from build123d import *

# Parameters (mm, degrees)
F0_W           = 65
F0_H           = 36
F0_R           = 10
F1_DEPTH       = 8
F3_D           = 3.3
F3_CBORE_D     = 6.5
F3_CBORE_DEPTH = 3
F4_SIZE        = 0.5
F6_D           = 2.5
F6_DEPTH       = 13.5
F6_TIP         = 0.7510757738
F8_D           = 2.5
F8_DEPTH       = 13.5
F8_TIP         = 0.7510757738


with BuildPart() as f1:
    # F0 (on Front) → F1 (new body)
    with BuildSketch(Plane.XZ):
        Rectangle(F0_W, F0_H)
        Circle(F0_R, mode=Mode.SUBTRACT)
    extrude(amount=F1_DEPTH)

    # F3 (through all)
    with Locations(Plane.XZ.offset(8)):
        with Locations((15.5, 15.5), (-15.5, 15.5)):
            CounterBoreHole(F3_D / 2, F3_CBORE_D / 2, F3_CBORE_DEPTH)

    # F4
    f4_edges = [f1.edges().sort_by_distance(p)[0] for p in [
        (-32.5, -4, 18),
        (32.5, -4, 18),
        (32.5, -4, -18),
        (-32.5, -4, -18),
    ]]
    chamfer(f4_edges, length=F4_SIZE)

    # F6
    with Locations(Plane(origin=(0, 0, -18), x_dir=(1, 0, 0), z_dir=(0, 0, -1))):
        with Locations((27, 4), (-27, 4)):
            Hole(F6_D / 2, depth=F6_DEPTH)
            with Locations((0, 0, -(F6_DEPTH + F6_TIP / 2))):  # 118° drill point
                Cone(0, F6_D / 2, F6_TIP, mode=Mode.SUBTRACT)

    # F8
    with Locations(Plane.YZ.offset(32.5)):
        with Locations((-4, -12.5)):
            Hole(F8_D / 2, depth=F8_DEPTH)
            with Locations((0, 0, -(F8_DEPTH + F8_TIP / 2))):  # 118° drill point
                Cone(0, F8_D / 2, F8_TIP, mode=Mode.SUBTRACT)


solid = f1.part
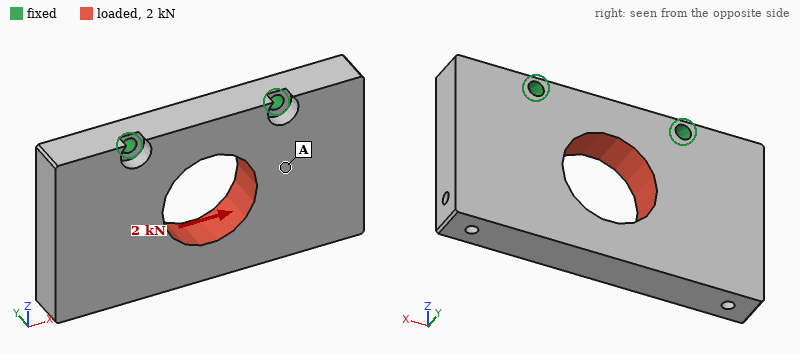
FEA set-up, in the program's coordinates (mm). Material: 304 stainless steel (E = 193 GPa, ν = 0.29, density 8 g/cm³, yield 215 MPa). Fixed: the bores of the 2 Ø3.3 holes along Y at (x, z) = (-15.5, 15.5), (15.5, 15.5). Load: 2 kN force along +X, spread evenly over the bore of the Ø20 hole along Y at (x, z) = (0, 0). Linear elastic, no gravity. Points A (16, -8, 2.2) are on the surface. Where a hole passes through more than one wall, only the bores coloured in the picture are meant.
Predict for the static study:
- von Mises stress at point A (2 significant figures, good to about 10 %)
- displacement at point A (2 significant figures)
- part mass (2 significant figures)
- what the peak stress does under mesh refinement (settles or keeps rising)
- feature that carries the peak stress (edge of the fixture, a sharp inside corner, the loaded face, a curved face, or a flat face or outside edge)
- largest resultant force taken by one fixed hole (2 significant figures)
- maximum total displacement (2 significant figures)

10 MPa
3.9 µm
130 g
keeps rising
edge of the fixture
1.3 kN
9.9 µm
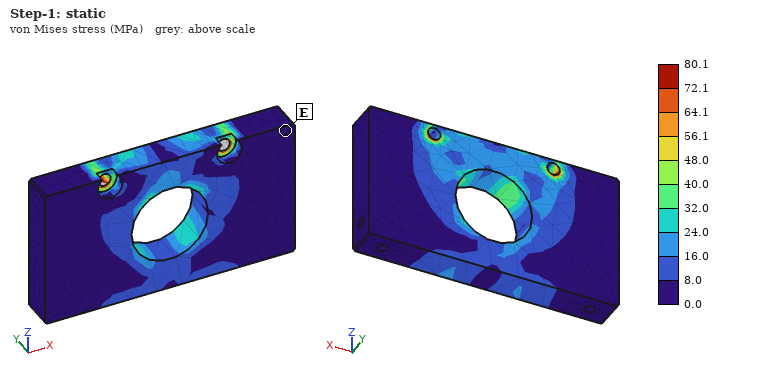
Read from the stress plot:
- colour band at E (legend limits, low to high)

0.0 to 8.0 MPa
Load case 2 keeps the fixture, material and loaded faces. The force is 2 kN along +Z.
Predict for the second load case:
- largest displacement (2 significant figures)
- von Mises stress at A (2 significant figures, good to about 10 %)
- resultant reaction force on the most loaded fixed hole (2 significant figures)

6.5 µm
7.5 MPa
1.0 kN
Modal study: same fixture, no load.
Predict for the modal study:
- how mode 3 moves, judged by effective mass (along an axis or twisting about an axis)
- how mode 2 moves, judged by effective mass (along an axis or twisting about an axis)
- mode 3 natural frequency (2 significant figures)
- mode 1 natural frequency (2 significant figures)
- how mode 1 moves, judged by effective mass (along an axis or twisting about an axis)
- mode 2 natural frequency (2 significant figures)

along X
twisting about Z
7200 Hz
2700 Hz
along Y
4600 Hz
